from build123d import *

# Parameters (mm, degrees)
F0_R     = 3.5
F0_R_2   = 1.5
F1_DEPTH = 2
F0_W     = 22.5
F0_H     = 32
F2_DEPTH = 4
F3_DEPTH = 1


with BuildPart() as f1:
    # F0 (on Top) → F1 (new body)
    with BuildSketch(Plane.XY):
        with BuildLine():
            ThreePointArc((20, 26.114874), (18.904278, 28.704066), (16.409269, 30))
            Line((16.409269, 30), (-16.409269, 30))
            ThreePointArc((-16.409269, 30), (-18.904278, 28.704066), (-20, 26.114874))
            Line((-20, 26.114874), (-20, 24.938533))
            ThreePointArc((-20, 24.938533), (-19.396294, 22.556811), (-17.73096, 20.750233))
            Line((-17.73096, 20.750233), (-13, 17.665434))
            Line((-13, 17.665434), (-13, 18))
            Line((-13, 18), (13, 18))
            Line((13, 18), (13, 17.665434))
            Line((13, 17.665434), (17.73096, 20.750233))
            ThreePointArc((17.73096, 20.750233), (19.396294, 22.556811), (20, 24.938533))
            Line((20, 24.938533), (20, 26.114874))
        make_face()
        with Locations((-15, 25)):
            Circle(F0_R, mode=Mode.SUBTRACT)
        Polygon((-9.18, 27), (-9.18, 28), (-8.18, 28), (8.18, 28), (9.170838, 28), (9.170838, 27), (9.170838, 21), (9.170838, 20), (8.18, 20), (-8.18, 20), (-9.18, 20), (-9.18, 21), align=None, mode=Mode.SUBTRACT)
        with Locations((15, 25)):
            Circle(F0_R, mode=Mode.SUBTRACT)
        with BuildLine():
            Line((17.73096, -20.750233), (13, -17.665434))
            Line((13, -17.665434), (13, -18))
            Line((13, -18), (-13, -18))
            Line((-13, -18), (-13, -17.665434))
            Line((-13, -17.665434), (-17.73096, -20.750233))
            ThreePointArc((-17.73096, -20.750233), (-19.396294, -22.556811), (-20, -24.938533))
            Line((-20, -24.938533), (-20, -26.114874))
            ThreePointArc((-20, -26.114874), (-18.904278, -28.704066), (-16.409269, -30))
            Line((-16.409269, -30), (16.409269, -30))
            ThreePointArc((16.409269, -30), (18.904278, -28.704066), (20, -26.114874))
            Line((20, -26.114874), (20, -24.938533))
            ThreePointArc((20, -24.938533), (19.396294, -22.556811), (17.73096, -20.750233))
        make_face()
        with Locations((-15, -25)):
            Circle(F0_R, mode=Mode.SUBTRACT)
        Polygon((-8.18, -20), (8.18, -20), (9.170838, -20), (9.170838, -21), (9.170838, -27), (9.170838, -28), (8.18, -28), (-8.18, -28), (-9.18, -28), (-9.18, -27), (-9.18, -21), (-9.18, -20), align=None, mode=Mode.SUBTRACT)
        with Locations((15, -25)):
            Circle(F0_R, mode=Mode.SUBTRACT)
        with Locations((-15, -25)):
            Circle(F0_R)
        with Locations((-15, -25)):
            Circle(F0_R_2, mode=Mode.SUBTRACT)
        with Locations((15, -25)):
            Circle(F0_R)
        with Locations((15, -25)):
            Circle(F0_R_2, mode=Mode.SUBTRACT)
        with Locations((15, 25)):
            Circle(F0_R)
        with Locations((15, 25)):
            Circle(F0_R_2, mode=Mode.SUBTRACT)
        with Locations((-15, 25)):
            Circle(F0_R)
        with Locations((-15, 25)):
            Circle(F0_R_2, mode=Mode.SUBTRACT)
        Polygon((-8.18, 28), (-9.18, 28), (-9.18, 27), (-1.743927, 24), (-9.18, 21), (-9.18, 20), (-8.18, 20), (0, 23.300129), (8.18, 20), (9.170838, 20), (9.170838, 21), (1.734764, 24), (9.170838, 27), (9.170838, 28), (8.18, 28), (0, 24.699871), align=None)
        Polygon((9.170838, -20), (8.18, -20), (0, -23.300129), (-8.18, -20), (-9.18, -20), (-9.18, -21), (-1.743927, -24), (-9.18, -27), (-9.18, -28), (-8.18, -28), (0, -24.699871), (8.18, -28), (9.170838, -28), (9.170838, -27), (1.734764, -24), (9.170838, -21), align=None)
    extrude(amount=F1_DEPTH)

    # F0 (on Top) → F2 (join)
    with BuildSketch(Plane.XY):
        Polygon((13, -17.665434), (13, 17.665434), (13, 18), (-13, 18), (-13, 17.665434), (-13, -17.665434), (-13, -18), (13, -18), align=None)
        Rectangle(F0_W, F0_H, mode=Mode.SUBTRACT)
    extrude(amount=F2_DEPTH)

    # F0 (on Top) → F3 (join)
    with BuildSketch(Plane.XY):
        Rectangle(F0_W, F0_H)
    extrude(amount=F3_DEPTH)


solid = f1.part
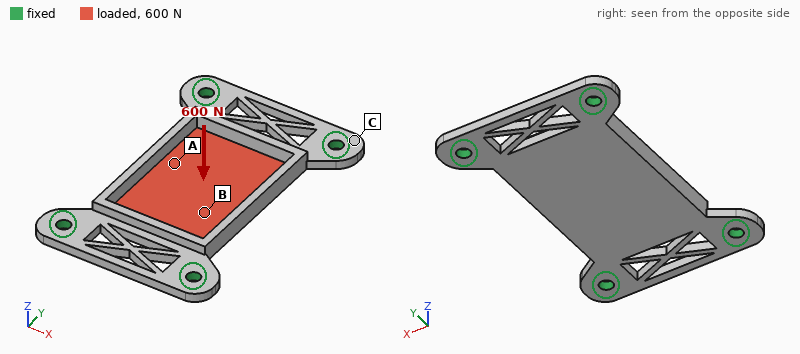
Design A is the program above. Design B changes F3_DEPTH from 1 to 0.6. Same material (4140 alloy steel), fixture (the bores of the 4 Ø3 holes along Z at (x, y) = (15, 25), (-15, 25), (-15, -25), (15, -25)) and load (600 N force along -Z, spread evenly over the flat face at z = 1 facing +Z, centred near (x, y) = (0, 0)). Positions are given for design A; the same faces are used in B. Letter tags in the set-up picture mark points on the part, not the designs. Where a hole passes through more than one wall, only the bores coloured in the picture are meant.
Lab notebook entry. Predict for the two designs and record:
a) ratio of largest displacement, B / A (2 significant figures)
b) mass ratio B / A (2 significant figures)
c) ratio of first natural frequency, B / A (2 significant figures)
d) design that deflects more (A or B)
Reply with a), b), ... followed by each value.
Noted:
a) 1.9
b) 0.90
c) 1.0
d) B
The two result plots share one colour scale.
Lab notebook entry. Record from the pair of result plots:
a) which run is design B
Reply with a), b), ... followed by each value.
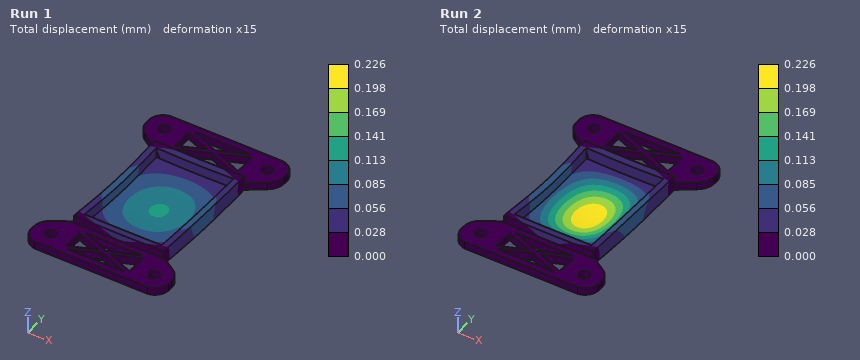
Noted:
a) Run 2
